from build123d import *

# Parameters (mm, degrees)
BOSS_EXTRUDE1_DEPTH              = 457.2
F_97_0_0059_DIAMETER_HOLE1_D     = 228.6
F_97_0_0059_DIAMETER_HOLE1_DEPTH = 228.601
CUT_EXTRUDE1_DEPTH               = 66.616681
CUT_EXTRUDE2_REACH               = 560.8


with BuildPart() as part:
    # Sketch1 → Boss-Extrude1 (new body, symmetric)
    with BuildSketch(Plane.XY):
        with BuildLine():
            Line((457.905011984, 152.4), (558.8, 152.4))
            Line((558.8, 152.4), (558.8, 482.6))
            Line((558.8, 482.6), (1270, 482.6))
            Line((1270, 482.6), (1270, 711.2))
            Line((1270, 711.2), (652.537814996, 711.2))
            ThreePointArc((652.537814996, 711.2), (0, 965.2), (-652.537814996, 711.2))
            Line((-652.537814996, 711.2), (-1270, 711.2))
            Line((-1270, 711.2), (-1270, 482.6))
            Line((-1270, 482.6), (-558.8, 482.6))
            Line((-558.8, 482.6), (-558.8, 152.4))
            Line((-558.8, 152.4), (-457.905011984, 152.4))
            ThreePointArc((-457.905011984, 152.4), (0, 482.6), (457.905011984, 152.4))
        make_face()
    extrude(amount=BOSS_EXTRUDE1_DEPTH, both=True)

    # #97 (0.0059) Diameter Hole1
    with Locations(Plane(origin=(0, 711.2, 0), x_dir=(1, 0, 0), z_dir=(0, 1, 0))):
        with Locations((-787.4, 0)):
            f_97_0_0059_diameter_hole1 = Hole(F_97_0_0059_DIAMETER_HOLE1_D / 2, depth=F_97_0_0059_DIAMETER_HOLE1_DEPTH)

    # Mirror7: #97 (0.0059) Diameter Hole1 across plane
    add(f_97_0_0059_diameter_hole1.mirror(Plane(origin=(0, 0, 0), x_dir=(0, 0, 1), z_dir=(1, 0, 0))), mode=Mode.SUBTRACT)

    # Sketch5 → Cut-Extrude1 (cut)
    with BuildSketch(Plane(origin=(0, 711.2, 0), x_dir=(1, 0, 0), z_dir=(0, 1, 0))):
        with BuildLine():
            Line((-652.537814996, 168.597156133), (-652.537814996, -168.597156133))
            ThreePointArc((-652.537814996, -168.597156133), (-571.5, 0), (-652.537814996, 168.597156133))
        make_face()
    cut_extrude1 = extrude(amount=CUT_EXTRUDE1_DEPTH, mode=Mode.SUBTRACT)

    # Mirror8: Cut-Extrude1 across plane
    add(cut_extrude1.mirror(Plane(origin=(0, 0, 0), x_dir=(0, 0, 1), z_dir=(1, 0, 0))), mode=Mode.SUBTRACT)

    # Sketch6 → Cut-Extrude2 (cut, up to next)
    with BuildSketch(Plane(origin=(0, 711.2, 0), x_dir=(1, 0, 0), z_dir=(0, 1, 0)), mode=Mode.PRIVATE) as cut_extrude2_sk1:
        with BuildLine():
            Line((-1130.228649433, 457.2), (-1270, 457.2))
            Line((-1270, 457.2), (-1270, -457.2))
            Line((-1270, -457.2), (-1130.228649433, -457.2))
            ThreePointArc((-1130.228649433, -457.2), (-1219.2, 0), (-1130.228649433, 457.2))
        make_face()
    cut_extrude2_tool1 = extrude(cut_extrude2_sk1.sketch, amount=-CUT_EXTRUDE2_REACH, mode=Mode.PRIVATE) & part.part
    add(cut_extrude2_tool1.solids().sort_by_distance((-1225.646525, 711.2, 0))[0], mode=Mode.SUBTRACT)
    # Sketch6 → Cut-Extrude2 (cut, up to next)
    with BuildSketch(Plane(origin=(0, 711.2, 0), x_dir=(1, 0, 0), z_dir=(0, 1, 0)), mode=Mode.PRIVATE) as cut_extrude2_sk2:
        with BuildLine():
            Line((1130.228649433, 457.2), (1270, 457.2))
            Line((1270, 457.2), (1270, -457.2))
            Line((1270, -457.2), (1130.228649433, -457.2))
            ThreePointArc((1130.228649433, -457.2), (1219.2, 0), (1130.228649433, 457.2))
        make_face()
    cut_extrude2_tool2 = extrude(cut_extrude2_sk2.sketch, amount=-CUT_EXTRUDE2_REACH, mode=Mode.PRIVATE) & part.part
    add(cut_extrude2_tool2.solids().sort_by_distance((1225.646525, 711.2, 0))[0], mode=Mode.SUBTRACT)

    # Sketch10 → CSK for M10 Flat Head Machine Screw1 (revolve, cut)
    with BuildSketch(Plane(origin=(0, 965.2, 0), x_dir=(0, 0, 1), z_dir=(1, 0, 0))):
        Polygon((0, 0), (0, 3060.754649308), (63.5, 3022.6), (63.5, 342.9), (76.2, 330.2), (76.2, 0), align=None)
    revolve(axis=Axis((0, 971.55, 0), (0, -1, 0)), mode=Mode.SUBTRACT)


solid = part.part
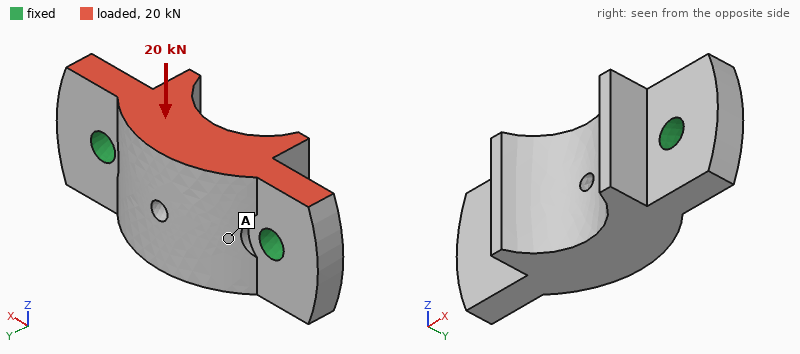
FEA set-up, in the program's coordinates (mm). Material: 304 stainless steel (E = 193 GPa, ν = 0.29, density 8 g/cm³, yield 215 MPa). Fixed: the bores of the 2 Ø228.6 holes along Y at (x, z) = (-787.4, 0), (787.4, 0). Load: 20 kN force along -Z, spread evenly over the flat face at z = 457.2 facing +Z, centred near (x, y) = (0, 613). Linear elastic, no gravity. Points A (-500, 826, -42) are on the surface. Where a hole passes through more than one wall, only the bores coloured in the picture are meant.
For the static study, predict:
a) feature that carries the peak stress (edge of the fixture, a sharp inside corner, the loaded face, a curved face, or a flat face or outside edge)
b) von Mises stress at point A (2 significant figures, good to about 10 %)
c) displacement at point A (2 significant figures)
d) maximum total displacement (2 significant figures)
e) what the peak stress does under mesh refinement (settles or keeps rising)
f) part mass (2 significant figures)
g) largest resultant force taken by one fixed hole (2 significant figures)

edge of the fixture
0.047 MPa
0.22 µm
0.42 µm
keeps rising
6500 kg
10 kN
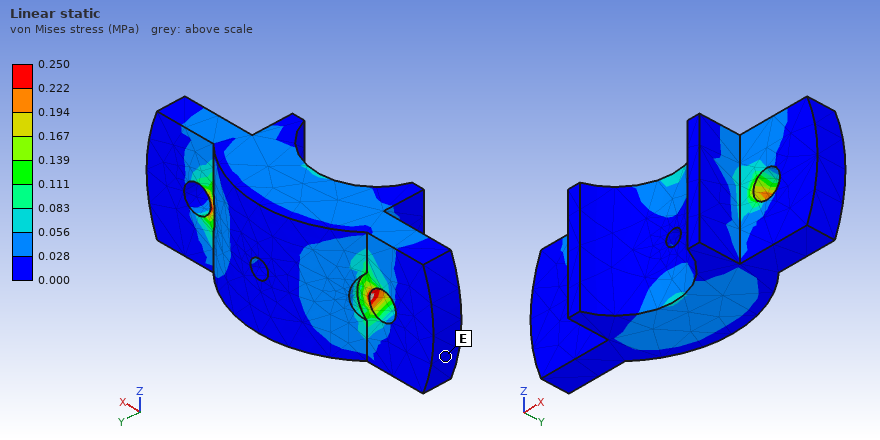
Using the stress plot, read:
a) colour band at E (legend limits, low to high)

0.000 to 0.028 MPa
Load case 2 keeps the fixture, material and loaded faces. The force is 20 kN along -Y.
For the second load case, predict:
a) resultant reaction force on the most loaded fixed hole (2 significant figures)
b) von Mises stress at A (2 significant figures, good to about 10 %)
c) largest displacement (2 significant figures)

10 kN
0.13 MPa
2.5 µm
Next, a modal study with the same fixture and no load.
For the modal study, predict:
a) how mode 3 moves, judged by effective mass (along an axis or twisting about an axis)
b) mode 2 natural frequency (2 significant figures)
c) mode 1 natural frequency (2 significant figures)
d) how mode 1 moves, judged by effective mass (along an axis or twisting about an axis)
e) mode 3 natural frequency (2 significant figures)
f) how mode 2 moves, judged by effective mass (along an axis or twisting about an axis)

along Z
440 Hz
340 Hz
twisting about X
560 Hz
along Y
